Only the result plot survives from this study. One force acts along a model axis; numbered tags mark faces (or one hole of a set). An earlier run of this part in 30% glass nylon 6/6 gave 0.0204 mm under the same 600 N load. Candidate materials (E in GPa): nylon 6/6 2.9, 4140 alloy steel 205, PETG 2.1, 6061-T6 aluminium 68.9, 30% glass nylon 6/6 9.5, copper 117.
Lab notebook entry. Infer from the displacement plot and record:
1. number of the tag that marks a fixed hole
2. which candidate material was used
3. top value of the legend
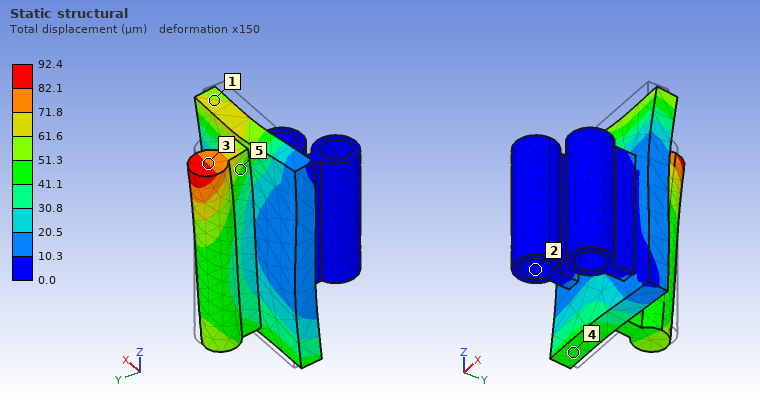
2
PETG
92.4 µm
